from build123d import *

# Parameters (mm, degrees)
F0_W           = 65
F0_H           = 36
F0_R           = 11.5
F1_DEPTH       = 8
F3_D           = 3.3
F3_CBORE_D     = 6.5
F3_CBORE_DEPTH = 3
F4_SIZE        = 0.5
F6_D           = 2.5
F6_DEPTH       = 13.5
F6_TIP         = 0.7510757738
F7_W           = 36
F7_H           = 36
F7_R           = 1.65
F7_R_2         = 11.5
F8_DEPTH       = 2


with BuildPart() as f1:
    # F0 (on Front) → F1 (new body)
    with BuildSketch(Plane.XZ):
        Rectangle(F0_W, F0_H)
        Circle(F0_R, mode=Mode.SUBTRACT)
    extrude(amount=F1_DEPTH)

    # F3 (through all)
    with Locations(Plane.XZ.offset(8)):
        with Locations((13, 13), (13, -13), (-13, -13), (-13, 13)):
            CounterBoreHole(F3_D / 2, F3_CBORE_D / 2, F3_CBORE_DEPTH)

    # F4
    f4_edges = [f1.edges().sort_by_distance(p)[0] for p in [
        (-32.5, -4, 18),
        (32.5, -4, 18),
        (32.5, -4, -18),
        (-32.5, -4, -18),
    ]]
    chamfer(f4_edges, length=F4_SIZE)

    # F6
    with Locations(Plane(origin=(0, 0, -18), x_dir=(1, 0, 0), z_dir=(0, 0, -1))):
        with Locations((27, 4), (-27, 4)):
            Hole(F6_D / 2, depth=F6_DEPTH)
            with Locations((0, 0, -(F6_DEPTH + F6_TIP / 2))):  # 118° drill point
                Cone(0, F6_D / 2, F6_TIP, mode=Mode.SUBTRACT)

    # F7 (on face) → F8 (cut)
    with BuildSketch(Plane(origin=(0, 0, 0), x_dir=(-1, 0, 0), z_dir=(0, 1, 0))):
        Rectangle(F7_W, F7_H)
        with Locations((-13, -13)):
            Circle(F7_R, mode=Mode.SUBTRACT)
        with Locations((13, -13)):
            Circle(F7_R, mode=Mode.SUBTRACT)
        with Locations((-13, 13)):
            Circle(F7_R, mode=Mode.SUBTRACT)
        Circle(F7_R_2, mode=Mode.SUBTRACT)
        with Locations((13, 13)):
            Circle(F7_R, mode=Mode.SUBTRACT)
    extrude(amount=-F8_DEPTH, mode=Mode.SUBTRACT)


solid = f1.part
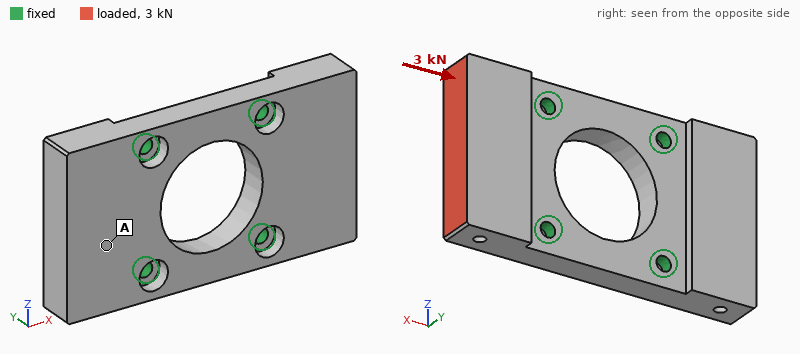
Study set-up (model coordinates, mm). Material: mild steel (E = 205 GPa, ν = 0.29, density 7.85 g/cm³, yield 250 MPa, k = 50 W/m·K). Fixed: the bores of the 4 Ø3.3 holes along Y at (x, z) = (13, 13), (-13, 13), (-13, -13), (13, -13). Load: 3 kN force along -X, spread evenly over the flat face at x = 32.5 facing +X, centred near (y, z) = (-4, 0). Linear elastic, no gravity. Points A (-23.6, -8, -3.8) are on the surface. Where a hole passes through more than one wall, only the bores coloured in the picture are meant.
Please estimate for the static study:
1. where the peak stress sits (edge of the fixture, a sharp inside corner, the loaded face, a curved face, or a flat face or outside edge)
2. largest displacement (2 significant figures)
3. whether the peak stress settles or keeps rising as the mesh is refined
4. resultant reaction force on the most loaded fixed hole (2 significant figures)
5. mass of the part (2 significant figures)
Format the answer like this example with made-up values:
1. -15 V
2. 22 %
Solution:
1. edge of the fixture
2. 2.3 µm
3. keeps rising
4. 1.4 kN
5. 100 g
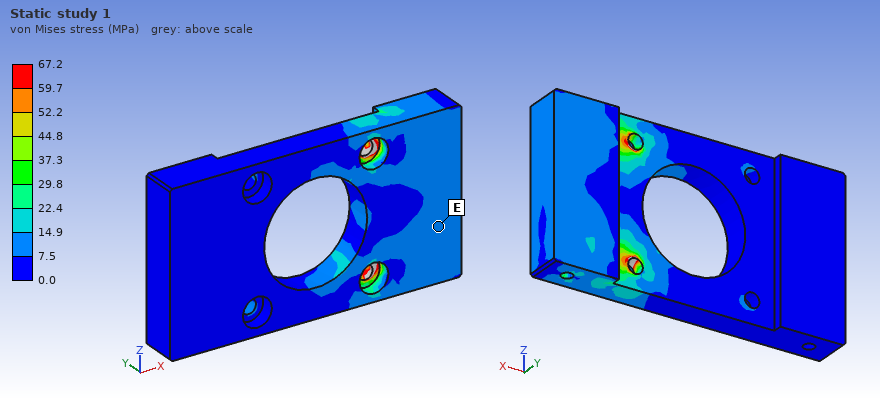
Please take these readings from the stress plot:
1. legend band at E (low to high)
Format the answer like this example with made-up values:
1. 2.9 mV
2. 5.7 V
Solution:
1. 7.5 to 14.9 MPa
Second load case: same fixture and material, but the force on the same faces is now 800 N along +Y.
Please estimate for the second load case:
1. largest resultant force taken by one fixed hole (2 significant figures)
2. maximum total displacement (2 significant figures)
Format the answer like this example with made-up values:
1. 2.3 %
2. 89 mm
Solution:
1. 620 N
2. 36 µm
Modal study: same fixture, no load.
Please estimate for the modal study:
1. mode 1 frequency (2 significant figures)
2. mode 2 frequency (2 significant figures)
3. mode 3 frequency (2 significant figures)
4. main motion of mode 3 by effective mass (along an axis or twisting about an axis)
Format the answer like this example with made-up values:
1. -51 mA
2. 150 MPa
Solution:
1. 6400 Hz
2. 6700 Hz
3. 16 kHz
4. twisting about X
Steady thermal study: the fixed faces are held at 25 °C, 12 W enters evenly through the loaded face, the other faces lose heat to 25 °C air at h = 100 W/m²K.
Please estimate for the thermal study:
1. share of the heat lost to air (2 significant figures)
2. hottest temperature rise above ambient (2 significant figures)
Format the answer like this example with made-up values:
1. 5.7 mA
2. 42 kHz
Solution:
1. 24 %
2. 22 K
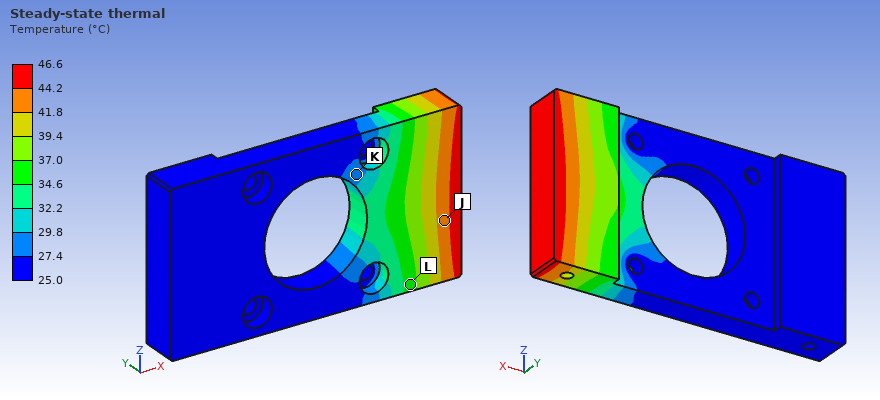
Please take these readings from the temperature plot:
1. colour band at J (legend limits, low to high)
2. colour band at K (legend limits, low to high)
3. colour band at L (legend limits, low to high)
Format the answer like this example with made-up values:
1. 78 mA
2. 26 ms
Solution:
1. 41.8 to 44.2 °C
2. 27.4 to 29.8 °C
3. 34.6 to 37.0 °C
